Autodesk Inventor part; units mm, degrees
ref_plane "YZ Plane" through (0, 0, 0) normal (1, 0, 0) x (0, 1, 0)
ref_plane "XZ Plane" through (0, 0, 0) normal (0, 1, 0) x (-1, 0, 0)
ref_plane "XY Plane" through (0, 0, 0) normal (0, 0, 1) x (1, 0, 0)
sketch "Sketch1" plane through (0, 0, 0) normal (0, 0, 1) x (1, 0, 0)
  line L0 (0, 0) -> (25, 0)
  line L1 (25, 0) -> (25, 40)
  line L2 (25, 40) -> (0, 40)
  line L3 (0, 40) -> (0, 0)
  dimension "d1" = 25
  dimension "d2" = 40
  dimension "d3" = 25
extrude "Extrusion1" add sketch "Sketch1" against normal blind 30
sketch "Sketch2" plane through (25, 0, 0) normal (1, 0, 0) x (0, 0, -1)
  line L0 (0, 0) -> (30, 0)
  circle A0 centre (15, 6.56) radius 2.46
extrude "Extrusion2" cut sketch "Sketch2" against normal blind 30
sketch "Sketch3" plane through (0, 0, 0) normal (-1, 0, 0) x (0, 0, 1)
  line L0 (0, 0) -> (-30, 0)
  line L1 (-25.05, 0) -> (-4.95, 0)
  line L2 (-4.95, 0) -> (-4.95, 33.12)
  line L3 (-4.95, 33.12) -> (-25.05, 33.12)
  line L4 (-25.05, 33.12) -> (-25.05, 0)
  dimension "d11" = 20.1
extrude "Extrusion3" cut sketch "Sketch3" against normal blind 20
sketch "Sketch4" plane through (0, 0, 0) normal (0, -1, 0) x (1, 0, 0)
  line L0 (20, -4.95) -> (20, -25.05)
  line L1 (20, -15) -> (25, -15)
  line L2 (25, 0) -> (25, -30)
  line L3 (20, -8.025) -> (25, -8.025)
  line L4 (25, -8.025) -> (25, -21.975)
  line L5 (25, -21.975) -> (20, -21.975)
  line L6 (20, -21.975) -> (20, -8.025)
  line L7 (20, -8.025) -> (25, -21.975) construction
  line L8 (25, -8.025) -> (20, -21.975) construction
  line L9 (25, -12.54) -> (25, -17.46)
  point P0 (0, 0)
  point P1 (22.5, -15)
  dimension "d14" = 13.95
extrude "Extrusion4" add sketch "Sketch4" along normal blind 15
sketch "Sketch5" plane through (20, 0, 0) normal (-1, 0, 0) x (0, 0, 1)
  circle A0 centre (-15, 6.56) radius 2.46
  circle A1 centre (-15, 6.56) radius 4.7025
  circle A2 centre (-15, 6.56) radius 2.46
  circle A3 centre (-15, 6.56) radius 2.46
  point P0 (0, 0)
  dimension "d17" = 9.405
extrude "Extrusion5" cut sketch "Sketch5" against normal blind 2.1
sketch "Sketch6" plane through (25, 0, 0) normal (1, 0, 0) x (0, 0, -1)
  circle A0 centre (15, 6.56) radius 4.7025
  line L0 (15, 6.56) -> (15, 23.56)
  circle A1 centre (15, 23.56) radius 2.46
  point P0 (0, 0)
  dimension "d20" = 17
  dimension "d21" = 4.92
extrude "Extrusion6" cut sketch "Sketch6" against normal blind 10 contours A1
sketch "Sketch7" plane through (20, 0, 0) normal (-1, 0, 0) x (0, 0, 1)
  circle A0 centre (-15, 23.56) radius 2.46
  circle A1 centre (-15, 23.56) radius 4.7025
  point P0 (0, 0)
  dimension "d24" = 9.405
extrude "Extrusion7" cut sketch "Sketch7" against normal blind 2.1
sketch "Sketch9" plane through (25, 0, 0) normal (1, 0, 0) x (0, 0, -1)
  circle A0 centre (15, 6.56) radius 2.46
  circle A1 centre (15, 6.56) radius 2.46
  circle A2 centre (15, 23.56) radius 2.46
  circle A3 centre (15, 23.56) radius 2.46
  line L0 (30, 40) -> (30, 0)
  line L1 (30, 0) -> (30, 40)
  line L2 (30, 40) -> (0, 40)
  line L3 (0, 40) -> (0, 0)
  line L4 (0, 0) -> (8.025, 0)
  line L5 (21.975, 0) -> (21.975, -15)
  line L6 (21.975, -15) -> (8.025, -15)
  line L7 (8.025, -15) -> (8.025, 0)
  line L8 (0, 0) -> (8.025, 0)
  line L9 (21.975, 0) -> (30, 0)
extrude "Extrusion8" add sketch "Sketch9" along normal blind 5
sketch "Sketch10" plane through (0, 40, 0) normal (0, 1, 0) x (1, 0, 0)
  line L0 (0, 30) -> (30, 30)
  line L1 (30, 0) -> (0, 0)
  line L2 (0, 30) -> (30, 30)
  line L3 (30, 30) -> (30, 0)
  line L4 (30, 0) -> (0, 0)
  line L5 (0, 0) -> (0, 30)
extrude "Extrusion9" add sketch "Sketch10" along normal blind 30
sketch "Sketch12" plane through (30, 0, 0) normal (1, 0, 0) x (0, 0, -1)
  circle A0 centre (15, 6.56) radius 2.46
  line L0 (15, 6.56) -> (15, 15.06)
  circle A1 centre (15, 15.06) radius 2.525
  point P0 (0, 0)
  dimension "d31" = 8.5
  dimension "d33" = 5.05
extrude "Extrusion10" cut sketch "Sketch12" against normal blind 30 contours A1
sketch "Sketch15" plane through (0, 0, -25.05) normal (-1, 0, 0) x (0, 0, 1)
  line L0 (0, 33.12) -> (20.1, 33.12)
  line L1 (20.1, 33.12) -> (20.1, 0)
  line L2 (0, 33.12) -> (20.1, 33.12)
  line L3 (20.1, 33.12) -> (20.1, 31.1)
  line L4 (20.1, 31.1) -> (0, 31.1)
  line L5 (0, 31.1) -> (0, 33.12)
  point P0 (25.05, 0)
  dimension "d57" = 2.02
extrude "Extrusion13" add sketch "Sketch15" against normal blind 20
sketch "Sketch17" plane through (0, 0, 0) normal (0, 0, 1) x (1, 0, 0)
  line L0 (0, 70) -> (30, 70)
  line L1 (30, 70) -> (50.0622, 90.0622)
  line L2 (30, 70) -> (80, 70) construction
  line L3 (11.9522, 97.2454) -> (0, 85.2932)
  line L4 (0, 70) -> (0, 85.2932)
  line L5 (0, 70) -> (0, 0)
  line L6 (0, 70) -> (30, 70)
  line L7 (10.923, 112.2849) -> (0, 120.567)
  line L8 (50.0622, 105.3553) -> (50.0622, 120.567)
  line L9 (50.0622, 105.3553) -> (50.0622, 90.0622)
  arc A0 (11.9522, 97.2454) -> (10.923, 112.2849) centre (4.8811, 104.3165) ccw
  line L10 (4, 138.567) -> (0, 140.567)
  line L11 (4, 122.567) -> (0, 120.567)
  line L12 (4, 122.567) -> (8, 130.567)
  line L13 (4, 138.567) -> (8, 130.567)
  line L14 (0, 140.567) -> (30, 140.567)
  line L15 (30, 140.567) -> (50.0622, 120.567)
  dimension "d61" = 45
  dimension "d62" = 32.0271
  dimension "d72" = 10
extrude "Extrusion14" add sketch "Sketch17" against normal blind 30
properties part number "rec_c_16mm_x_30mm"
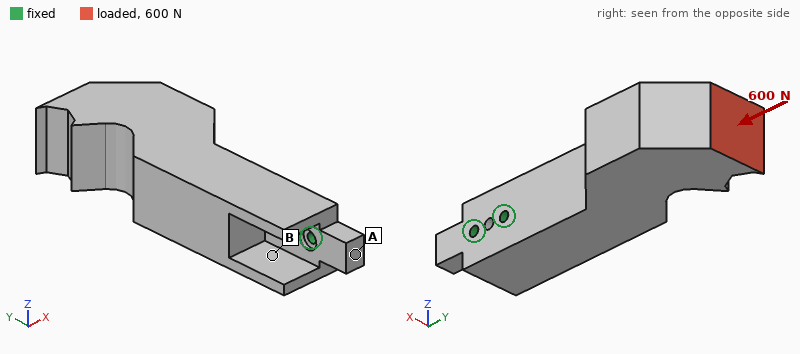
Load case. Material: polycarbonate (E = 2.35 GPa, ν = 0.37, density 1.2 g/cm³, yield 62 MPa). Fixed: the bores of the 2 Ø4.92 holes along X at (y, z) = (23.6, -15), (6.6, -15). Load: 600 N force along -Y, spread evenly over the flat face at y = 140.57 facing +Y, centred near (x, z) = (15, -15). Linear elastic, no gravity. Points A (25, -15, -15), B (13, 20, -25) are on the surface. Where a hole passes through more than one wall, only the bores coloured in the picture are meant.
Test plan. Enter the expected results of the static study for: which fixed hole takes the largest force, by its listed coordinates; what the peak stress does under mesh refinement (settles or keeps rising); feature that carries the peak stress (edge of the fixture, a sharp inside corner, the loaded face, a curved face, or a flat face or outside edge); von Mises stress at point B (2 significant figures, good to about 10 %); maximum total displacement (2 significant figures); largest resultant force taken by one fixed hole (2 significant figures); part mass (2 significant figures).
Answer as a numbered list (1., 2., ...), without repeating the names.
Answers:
1. (23.6, -15)
2. keeps rising
3. edge of the fixture
4. 2.3 MPa
5. 0.62 mm
6. 450 N
7. 160 g
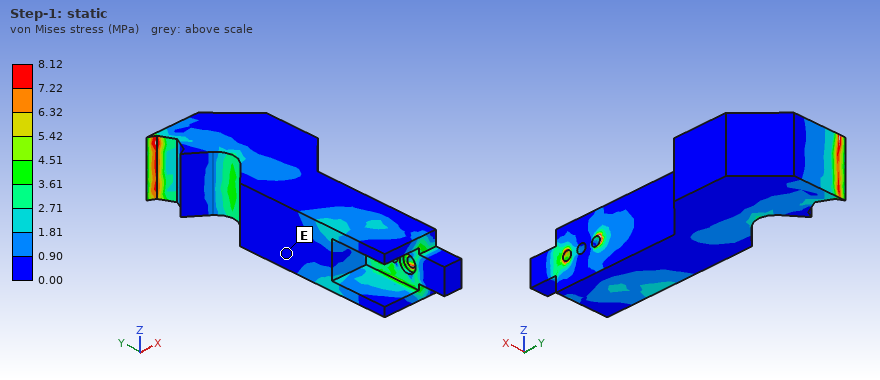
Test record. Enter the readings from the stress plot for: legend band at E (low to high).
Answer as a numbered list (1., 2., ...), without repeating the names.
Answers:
1. 0.00 to 0.90 MPa
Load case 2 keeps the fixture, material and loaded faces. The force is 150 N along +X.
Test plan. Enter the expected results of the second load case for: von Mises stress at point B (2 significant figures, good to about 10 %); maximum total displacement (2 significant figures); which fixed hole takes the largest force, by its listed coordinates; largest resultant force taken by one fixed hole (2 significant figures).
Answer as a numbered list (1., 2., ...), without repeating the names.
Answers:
1. 5.8 MPa
2. 1.8 mm
3. (23.6, -15)
4. 850 N
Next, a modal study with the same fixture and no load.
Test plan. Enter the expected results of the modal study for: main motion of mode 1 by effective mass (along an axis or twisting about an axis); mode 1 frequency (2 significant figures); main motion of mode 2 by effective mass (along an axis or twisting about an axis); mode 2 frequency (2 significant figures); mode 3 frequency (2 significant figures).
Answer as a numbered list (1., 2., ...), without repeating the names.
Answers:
1. along X
2. 210 Hz
3. along Z
4. 240 Hz
5. 650 Hz
